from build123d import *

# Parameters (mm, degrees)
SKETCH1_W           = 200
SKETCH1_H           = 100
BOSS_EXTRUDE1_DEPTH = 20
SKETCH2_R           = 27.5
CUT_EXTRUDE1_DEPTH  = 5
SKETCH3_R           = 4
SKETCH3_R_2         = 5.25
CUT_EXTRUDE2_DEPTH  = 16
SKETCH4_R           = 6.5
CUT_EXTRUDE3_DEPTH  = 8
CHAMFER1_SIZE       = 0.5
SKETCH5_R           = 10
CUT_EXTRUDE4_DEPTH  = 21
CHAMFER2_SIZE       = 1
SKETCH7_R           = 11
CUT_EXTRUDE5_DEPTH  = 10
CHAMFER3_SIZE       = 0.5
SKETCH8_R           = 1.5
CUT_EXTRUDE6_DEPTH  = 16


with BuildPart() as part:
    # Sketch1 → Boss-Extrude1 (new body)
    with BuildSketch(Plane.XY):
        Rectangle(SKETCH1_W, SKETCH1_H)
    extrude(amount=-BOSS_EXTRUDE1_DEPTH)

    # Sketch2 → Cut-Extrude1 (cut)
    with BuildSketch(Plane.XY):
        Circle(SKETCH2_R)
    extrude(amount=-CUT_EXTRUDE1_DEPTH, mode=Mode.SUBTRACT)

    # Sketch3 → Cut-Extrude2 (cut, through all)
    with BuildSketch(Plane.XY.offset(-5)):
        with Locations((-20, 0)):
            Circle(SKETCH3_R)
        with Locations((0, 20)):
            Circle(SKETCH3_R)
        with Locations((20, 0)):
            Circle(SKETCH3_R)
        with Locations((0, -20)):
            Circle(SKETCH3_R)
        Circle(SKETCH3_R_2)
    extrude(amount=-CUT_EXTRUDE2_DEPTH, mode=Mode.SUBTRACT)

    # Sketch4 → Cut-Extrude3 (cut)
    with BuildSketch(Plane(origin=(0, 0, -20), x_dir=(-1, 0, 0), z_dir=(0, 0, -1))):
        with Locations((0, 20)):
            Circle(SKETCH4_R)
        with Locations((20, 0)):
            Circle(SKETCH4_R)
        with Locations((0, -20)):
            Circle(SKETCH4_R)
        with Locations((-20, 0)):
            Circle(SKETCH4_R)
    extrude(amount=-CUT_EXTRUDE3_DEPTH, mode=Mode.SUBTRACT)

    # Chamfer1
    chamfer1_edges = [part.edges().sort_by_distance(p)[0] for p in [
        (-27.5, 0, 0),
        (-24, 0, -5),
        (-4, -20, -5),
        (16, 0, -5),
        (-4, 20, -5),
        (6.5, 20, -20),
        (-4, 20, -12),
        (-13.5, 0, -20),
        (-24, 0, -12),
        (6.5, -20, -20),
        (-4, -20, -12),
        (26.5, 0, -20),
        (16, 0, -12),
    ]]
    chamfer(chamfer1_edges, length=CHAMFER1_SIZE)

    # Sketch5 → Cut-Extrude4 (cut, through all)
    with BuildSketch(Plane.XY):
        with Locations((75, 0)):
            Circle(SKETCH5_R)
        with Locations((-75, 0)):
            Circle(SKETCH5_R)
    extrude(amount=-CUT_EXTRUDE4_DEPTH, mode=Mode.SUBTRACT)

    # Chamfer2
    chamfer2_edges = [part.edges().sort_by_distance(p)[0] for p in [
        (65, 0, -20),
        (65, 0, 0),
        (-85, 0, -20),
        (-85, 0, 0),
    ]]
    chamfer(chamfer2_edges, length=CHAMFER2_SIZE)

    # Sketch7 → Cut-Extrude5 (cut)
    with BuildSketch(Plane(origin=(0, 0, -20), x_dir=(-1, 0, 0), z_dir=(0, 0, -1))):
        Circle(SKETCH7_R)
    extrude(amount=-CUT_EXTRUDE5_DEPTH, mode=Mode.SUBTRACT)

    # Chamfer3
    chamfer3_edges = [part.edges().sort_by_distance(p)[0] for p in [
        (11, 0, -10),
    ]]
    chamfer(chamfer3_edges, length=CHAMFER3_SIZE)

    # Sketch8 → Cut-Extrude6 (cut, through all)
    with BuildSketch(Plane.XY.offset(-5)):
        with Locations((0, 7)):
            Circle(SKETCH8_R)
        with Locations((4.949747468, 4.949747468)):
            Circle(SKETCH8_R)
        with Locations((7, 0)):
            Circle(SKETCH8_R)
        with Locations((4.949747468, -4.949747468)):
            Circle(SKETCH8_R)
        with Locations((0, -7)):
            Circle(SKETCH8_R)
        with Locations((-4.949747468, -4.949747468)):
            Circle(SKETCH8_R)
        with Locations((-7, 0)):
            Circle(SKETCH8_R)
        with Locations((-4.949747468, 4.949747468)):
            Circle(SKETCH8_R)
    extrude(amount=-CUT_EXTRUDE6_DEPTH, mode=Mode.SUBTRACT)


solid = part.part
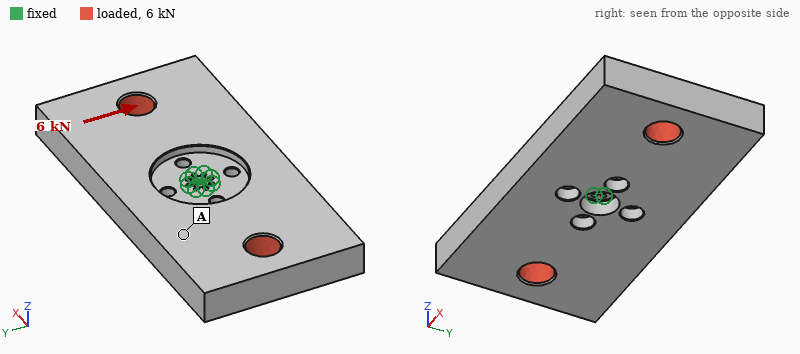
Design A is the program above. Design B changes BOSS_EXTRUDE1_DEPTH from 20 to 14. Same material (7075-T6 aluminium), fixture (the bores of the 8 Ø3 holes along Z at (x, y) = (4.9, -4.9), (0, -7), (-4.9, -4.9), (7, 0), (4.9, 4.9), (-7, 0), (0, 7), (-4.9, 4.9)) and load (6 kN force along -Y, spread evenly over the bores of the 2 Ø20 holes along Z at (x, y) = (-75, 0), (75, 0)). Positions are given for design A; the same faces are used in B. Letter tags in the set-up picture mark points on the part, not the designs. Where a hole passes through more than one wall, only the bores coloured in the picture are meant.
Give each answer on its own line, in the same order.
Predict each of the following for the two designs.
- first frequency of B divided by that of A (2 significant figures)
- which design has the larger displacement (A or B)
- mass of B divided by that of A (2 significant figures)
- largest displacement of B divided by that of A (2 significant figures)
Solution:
0.94
A
0.70
0.86
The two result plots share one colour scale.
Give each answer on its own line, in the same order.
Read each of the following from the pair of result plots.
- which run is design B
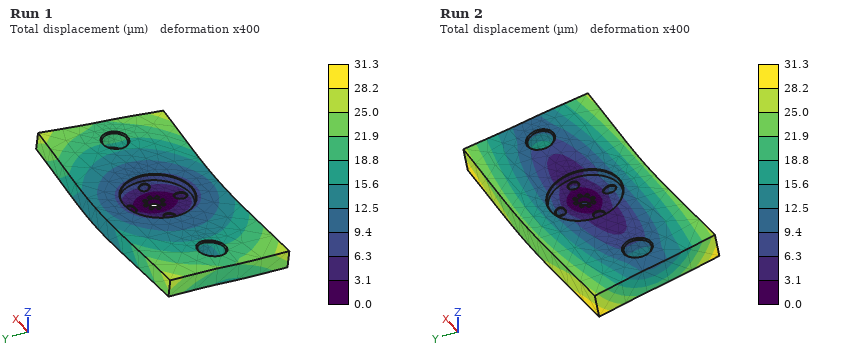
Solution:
Run 1
